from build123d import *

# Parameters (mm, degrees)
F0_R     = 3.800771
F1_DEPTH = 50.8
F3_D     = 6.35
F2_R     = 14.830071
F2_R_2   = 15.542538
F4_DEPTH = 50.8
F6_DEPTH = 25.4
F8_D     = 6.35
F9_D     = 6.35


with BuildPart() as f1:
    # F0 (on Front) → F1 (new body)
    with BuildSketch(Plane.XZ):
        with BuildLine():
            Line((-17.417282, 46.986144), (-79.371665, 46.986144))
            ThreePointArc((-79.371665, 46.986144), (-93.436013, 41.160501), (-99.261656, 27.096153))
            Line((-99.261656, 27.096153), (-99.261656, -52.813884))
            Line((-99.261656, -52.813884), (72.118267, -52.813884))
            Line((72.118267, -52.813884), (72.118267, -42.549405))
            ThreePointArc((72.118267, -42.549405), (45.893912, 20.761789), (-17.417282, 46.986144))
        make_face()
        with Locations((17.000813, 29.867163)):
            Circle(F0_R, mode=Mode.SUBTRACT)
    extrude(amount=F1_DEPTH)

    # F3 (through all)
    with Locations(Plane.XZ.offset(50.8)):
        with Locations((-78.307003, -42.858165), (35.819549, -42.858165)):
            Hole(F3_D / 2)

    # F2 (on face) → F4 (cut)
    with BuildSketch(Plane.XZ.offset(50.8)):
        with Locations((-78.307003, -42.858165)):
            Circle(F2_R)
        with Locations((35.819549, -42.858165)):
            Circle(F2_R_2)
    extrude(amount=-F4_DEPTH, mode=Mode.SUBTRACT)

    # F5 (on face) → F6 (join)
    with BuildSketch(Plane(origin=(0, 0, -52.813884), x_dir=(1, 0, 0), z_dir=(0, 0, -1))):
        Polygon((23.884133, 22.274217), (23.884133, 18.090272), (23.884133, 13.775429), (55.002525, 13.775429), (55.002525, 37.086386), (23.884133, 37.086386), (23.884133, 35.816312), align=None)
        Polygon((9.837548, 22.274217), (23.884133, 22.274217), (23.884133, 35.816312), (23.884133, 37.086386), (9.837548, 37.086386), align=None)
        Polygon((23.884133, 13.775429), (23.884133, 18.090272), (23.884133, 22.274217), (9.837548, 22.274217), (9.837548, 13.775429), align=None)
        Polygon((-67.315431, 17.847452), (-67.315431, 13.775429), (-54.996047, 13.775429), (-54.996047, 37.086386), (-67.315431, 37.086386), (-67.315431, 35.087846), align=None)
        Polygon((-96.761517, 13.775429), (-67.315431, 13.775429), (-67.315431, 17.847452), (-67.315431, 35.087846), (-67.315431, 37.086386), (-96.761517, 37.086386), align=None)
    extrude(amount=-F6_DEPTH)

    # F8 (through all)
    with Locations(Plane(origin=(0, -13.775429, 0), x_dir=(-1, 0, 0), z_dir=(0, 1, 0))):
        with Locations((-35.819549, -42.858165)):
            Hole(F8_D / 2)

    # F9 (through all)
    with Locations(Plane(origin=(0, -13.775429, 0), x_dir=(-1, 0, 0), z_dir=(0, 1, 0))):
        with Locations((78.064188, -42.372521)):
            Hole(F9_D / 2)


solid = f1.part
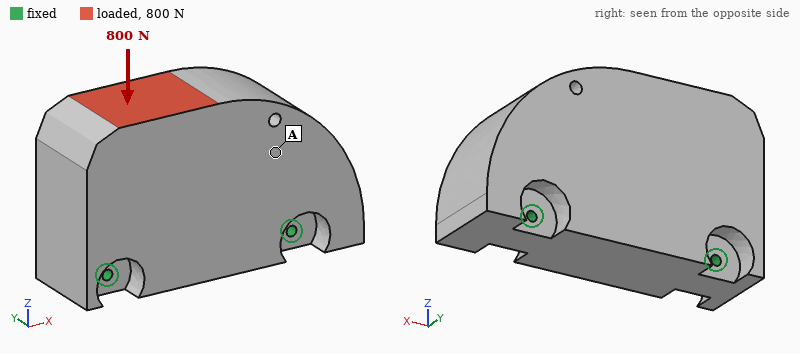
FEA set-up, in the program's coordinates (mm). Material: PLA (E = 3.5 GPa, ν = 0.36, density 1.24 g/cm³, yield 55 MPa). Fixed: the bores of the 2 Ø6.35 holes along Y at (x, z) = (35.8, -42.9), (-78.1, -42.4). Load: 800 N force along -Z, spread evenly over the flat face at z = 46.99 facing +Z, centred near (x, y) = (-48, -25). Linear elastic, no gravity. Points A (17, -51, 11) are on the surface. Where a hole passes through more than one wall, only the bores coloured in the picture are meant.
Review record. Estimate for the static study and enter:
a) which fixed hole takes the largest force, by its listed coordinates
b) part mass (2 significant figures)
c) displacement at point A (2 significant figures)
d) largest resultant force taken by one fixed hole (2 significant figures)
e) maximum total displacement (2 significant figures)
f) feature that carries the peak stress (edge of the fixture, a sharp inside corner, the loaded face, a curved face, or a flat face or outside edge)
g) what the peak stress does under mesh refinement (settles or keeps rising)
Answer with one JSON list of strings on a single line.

["(-78.1, -42.4)", "920 g", "4.1 µm", "600 N", "11 µm", "edge of the fixture", "keeps rising"]
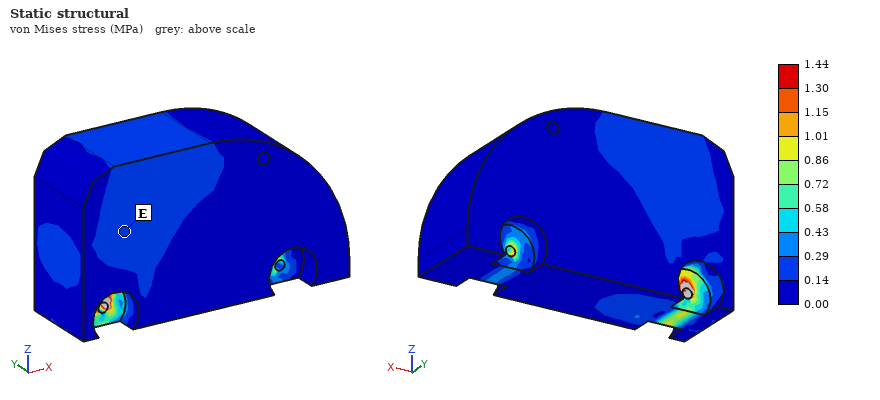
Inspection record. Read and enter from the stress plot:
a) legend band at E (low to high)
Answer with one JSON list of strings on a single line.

["0.14 to 0.29 MPa"]
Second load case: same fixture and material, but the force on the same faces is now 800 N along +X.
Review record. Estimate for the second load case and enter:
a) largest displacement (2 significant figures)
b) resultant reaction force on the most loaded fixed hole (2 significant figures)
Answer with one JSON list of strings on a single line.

["28 µm", "760 N"]
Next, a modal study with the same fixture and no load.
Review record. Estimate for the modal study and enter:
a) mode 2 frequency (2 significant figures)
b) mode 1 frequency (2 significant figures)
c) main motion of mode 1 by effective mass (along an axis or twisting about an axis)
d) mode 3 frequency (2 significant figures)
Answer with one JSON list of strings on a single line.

["1500 Hz", "420 Hz", "along Y", "1500 Hz"]
